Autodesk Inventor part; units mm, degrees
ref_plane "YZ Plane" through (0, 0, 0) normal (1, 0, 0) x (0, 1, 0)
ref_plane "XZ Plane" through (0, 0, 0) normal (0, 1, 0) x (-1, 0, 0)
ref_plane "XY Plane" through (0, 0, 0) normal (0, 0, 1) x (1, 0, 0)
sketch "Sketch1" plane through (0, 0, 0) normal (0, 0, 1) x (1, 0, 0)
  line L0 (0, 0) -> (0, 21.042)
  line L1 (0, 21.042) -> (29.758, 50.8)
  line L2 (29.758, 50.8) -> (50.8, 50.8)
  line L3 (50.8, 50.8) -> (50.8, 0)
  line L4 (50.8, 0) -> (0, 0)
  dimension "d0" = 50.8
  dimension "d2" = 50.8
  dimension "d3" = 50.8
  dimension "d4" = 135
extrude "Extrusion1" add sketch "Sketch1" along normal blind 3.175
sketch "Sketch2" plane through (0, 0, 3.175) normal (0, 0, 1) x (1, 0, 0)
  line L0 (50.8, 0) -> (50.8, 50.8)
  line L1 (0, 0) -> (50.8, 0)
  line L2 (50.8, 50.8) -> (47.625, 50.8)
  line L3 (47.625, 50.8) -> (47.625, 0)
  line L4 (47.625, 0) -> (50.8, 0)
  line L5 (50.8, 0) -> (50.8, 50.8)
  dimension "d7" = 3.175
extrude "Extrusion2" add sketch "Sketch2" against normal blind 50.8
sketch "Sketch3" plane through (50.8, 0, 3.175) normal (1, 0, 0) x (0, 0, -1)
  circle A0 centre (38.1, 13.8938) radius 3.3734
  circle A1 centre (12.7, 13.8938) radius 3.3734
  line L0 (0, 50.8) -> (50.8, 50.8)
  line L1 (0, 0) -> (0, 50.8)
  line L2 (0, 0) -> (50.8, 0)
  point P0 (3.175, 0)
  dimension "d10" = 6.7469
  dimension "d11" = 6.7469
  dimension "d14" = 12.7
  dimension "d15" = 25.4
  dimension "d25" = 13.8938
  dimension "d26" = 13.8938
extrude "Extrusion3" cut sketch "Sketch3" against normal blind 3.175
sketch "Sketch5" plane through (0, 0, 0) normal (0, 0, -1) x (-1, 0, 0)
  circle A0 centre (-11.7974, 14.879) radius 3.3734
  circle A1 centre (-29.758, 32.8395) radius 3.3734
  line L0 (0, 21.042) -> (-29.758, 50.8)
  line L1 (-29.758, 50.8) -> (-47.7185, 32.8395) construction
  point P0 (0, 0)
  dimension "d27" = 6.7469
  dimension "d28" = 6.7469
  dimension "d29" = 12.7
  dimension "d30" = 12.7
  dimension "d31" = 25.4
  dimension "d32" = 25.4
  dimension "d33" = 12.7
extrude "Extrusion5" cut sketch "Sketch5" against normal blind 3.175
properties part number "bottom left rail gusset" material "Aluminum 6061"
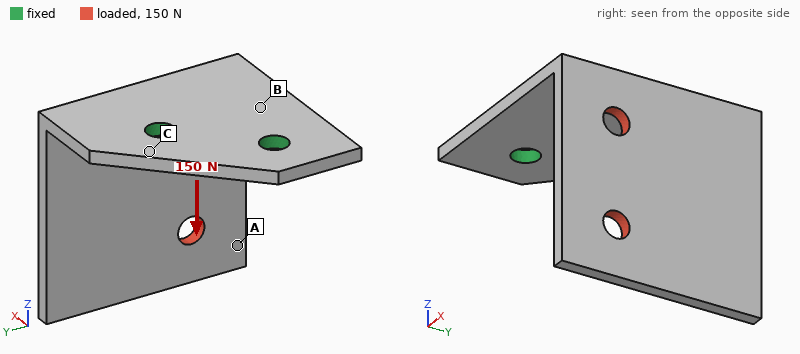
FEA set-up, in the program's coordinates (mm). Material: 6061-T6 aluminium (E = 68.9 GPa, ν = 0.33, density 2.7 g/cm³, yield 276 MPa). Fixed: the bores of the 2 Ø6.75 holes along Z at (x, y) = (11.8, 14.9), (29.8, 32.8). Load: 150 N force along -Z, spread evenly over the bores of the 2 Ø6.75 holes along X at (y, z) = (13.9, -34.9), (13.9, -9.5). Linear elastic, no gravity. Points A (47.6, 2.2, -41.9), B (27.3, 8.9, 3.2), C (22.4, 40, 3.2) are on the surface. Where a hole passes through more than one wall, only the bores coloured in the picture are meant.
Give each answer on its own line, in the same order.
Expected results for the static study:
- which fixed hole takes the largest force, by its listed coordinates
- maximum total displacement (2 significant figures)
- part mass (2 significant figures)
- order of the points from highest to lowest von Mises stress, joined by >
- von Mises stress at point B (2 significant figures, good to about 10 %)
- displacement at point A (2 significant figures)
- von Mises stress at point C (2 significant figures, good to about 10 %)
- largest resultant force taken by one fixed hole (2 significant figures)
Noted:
(29.8, 32.8)
0.28 mm
38 g
B > C > A
21 MPa
0.25 mm
12 MPa
140 N
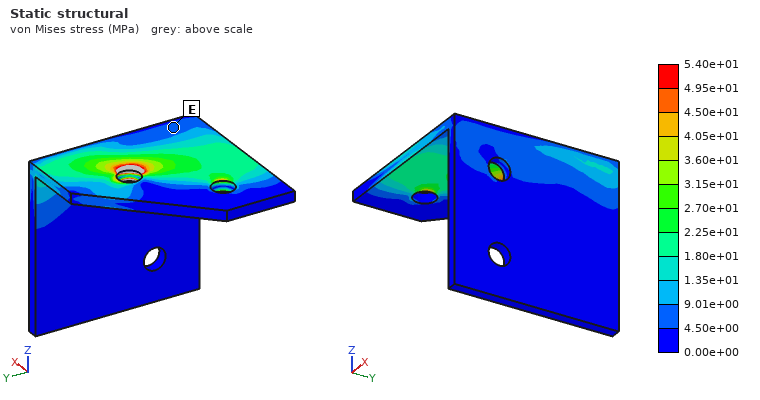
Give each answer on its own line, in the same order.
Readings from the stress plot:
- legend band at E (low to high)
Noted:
4.50e+00 to 9.01e+00 MPa
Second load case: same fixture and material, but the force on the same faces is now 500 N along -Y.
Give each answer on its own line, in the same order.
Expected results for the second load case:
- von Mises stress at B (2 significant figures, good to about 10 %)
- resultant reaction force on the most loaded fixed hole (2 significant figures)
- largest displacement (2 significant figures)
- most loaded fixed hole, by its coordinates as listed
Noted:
61 MPa
670 N
0.76 mm
(29.8, 32.8)
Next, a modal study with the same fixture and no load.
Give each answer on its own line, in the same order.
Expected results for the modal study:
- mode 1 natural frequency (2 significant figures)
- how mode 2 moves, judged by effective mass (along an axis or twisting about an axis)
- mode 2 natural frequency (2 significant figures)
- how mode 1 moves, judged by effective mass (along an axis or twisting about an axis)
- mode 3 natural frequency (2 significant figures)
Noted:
660 Hz
along Y
1000 Hz
along X
2300 Hz
